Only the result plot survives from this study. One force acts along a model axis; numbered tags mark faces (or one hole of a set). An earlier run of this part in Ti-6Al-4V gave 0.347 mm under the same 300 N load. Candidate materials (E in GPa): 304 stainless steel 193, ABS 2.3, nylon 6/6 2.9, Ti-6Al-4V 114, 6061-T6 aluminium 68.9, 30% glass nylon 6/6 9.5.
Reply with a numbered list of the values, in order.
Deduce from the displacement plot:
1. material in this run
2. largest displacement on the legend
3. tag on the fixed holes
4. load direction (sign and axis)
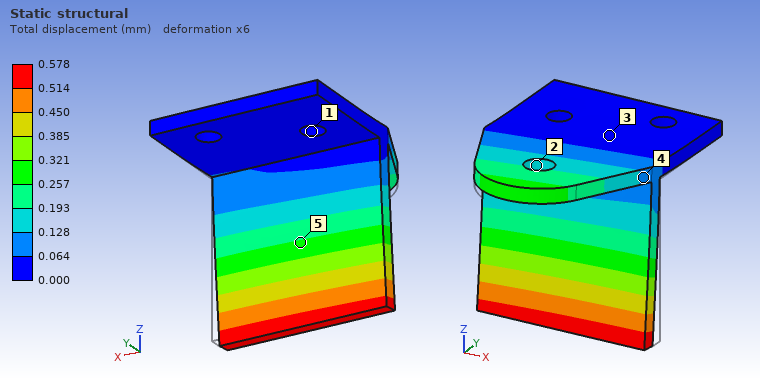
1. 6061-T6 aluminium
2. 0.578 mm
3. 1
4. -Y
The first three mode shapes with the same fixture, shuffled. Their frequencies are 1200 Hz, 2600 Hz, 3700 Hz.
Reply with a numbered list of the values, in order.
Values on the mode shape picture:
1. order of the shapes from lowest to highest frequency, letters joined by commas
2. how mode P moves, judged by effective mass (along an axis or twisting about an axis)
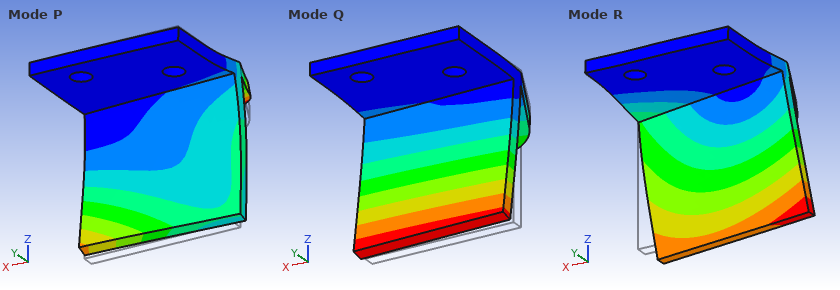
1. Q, R, P
2. along Z
